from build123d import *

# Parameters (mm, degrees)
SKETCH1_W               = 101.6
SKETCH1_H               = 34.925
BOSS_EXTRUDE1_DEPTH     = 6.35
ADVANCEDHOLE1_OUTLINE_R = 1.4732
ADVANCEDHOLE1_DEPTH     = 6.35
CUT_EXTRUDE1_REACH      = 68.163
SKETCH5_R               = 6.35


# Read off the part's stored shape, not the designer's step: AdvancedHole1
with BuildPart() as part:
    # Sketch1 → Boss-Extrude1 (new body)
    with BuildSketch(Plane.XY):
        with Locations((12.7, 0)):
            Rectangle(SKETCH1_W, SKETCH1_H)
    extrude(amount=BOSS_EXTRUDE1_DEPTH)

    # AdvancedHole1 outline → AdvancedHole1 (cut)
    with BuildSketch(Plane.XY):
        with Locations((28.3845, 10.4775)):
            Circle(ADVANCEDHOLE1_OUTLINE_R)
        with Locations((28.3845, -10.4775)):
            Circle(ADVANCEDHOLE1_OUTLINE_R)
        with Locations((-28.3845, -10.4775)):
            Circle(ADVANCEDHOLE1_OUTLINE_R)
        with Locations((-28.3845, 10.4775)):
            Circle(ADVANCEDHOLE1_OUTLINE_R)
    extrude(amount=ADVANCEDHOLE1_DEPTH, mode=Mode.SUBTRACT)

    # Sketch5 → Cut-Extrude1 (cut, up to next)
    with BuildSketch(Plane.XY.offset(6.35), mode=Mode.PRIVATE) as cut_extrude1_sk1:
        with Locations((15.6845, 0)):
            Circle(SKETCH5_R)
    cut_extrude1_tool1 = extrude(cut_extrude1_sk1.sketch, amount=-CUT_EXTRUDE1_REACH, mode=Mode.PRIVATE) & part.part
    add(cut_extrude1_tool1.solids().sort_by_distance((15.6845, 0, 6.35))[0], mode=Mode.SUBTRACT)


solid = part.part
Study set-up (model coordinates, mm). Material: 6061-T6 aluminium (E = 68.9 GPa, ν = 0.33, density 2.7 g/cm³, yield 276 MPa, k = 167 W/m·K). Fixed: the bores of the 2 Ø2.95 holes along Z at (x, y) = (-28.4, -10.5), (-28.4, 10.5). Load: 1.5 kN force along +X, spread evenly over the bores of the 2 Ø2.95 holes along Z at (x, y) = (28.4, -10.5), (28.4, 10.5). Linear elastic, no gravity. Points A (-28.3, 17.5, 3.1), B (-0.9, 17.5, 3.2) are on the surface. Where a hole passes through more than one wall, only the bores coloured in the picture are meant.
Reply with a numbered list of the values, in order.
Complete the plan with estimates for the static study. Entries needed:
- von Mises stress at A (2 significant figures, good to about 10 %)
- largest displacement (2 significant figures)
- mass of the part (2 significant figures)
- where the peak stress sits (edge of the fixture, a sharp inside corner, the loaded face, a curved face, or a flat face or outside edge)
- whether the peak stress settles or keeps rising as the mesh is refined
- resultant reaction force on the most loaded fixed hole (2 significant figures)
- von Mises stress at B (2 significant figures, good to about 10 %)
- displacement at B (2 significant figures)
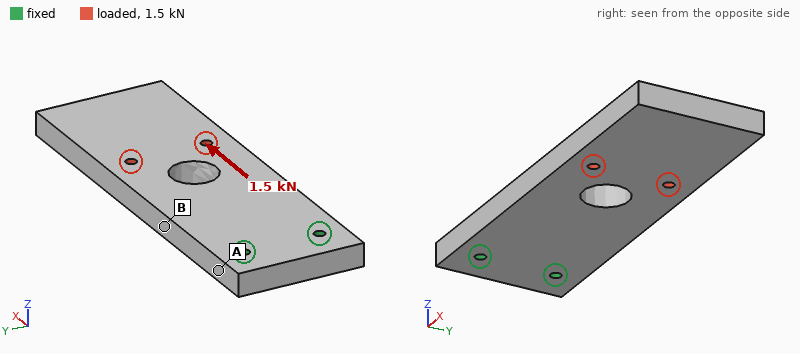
1. 4.3 MPa
2. 7.9 µm
3. 58 g
4. edge of the fixture
5. keeps rising
6. 750 N
7. 8.9 MPa
8. 3.4 µm
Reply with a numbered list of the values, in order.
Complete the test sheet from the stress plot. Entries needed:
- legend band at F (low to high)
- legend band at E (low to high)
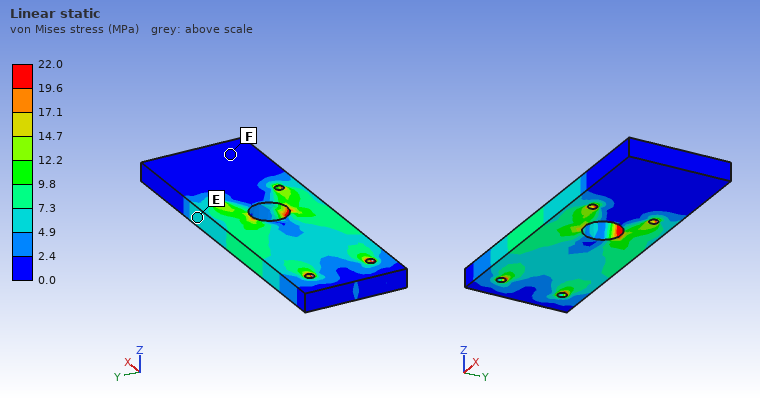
1. 0.0 to 2.4 MPa
2. 4.9 to 7.3 MPa
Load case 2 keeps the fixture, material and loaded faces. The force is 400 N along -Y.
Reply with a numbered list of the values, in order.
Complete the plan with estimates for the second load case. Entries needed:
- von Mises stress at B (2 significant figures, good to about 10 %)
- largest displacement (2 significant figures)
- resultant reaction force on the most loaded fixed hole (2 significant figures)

1. 10 MPa
2. 44 µm
3. 1.0 kN
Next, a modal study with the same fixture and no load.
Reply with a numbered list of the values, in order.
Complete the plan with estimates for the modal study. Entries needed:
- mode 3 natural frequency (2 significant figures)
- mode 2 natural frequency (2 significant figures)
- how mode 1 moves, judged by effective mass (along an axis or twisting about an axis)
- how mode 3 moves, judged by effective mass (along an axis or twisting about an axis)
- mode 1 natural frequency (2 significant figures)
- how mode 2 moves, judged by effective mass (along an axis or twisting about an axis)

1. 2900 Hz
2. 2800 Hz
3. along Z
4. twisting about X
5. 590 Hz
6. along Y
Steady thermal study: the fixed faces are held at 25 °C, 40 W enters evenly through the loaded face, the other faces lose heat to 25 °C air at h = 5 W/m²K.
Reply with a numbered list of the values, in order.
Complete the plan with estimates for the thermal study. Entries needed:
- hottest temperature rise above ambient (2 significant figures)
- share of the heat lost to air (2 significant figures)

1. 72 K
2. 4.6 %
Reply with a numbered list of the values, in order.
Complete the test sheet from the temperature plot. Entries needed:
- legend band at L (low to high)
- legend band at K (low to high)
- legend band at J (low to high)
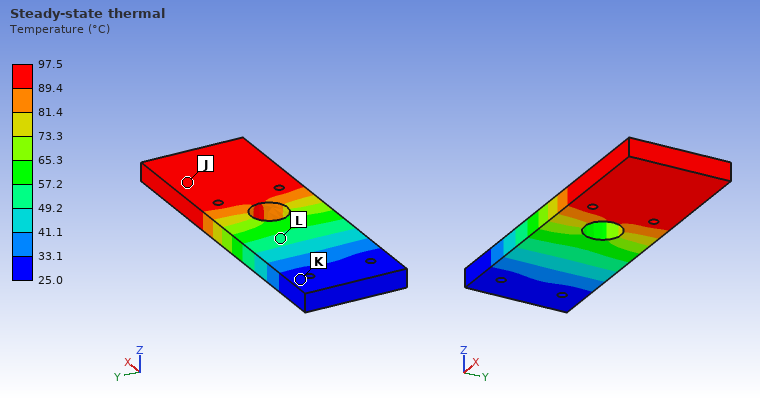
1. 49.2 to 57.2 °C
2. 25.0 to 33.1 °C
3. 89.4 to 97.5 °C
